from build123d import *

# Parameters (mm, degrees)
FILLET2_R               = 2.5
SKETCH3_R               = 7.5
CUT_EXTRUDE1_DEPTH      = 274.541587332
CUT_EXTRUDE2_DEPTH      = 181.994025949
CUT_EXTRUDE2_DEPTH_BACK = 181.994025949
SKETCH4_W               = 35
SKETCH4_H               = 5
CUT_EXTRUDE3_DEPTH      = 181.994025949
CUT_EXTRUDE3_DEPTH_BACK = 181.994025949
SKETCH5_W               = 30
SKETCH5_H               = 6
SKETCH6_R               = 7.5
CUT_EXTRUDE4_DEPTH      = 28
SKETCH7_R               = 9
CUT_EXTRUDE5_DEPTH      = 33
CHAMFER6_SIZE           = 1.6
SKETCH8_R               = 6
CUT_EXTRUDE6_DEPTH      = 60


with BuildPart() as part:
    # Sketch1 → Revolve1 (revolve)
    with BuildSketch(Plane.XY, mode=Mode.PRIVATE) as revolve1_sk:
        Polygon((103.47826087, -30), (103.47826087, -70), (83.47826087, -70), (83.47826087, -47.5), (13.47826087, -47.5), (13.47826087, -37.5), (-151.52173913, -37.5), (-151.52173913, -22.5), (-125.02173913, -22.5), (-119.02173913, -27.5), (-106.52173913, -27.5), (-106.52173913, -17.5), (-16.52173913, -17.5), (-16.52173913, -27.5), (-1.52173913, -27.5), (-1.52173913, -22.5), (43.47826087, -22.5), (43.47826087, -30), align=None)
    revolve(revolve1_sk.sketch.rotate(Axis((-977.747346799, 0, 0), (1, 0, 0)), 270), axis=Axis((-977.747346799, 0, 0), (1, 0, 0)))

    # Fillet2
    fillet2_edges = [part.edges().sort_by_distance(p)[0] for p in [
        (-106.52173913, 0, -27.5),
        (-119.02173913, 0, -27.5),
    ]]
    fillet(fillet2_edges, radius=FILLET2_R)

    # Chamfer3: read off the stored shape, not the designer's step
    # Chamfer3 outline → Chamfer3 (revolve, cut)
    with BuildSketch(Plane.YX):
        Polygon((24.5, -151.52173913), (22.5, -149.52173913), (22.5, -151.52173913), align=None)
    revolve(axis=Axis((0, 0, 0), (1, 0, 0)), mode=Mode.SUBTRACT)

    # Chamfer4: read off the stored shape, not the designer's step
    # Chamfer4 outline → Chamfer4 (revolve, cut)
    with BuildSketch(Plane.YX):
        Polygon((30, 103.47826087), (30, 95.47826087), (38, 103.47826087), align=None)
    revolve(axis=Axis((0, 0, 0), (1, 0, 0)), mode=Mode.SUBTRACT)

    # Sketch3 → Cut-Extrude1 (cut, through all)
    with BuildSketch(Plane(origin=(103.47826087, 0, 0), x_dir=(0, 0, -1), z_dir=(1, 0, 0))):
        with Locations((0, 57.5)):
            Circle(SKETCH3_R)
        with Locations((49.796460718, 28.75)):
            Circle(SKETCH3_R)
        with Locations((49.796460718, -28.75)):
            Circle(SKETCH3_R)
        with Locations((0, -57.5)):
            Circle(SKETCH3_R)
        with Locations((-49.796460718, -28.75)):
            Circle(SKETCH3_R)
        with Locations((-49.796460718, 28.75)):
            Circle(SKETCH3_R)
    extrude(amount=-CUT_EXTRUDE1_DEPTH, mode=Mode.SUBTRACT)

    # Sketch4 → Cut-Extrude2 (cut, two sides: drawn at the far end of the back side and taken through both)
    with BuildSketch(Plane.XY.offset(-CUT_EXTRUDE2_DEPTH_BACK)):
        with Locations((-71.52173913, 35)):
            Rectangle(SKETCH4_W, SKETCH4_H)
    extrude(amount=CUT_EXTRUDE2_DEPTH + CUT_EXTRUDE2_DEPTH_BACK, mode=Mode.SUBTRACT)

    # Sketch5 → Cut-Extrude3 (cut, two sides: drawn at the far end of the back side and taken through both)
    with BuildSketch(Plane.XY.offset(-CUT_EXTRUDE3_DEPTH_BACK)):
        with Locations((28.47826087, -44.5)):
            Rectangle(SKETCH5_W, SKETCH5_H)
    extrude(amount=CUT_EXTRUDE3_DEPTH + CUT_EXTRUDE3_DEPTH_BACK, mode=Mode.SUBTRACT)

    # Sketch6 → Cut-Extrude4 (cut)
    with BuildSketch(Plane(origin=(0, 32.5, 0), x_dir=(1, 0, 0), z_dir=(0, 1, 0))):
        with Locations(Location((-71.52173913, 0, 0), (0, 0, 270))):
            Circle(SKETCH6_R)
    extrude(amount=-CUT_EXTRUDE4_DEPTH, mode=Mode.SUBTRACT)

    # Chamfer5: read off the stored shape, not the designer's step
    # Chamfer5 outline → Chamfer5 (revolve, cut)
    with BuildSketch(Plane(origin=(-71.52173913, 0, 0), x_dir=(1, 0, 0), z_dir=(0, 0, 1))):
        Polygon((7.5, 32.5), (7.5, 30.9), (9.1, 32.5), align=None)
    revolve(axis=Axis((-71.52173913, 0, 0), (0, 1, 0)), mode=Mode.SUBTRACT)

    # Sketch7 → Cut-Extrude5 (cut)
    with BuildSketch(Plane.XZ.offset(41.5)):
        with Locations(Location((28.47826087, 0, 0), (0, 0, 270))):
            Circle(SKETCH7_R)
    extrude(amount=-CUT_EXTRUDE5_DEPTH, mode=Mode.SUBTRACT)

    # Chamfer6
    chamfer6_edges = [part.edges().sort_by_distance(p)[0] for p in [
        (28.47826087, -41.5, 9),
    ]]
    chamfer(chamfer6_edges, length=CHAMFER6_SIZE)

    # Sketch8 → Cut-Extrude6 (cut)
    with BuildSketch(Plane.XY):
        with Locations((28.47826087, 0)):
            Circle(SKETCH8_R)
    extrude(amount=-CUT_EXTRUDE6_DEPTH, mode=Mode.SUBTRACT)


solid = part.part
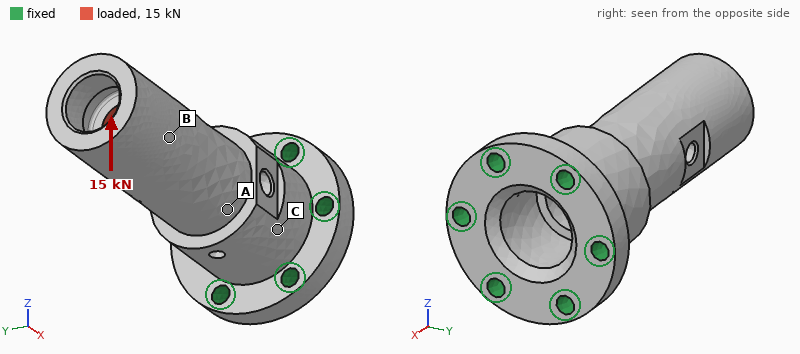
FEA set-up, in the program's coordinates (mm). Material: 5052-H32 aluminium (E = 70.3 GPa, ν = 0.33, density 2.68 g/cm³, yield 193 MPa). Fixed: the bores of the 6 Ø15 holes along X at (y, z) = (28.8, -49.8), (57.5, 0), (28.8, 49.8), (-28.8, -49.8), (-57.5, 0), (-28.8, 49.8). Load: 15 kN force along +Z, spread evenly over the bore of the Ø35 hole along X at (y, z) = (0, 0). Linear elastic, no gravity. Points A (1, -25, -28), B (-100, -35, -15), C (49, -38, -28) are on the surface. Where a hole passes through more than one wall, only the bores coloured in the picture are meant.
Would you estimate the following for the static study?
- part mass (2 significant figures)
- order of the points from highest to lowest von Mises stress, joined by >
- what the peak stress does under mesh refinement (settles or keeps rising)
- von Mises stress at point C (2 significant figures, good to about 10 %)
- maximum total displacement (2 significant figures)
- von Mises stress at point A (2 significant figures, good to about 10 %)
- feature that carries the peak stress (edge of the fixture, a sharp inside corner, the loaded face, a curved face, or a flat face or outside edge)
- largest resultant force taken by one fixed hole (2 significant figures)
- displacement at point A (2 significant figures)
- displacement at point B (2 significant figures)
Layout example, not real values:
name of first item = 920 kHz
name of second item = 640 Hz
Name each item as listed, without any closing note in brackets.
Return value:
part mass = 2.8 kg
order of the points from highest to lowest von Mises stress, joined by > = A > C > B
what the peak stress does under mesh refinement = keeps rising
von Mises stress at point C = 13 MPa
maximum total displacement = 0.28 mm
von Mises stress at point A = 28 MPa
feature that carries the peak stress = edge of the fixture
largest resultant force taken by one fixed hole = 14 kN
displacement at point A = 0.072 mm
displacement at point B = 0.21 mm
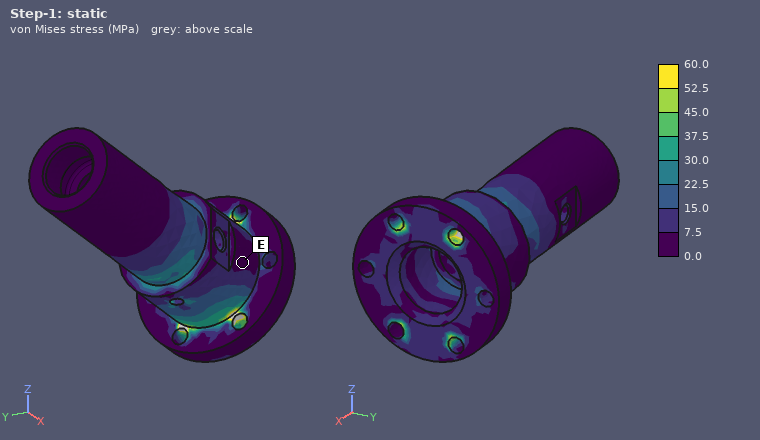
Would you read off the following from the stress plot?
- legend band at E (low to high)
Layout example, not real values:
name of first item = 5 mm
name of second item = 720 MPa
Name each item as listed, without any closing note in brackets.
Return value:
legend band at E = 0.0 to 7.5 MPa
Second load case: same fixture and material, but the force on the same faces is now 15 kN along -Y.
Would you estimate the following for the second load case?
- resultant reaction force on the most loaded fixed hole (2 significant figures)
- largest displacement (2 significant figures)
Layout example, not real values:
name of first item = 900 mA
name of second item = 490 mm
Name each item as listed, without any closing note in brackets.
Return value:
resultant reaction force on the most loaded fixed hole = 16 kN
largest displacement = 0.29 mm
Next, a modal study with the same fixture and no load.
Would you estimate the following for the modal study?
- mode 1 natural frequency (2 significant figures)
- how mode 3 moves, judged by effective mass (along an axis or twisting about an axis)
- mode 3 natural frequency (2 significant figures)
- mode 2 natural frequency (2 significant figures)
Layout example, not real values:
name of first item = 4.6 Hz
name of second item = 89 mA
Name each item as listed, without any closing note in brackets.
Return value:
mode 1 natural frequency = 1100 Hz
how mode 3 moves, judged by effective mass = twisting about X
mode 3 natural frequency = 3800 Hz
mode 2 natural frequency = 1200 Hz
